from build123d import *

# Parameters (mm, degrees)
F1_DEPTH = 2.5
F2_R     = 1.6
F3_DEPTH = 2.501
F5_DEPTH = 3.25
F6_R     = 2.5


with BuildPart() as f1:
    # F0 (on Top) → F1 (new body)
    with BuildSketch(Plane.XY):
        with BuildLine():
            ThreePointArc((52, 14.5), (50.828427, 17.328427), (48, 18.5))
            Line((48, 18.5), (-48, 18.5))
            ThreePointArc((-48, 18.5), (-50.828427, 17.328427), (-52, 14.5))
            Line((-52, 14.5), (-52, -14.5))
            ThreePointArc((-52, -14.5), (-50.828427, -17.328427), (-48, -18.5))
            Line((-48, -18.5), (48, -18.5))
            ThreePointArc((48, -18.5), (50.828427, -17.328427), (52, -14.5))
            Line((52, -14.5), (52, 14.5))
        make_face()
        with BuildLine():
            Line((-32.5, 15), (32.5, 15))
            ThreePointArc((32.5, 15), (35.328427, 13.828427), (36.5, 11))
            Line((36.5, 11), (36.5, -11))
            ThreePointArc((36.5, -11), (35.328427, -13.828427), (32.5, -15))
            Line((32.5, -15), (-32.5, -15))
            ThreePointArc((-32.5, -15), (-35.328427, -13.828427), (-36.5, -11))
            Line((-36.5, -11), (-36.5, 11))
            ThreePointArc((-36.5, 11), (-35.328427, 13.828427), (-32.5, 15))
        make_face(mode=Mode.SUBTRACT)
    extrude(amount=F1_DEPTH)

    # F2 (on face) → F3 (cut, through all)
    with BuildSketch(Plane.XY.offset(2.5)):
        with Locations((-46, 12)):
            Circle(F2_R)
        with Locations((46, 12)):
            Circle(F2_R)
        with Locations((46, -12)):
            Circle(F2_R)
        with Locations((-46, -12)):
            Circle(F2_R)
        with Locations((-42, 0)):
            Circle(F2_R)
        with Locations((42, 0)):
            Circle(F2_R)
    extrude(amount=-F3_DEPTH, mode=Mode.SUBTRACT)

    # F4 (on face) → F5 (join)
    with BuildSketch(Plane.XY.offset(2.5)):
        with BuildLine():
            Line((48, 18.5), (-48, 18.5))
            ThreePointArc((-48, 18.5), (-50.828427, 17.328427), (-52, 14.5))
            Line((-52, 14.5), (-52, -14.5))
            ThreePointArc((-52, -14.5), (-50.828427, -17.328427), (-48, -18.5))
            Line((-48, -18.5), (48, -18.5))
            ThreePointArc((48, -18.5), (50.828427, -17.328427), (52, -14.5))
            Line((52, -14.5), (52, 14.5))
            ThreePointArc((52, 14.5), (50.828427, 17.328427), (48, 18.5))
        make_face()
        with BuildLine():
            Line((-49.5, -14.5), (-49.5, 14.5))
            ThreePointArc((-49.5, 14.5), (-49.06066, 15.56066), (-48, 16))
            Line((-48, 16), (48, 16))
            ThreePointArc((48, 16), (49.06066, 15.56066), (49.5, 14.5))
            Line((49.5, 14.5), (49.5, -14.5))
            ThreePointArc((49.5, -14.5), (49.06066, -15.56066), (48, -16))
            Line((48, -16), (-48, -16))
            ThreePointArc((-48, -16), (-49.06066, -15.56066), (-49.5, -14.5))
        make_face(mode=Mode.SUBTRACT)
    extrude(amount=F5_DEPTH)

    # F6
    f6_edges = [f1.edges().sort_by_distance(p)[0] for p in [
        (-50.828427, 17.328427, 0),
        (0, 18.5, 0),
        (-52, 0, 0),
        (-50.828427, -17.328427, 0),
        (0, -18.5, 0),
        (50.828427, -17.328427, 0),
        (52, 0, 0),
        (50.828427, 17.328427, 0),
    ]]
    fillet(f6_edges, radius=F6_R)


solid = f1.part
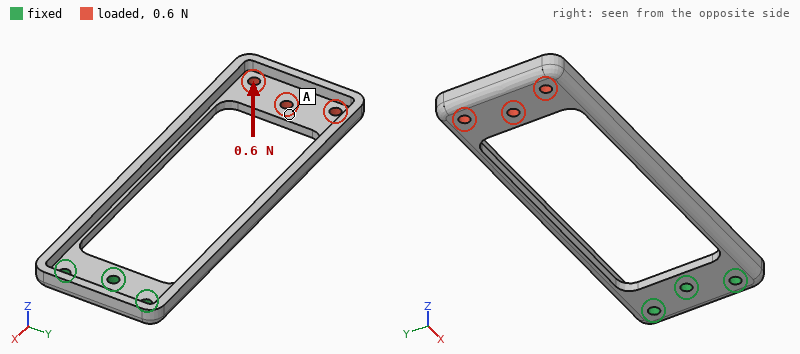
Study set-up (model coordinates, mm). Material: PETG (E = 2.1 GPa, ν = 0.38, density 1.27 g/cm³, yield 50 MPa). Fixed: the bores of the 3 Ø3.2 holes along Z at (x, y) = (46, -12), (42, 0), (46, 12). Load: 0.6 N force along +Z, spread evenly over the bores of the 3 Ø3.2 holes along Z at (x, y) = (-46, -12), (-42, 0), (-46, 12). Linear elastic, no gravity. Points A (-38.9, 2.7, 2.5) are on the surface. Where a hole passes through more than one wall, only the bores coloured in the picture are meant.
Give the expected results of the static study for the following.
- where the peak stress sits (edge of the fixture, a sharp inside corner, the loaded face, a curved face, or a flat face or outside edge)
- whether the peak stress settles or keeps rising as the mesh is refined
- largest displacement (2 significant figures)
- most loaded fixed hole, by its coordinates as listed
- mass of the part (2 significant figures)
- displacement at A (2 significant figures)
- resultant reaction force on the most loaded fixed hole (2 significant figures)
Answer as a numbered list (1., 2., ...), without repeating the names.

1. edge of the fixture
2. keeps rising
3. 1.0 mm
4. (42, 0)
5. 7.4 g
6. 0.82 mm
7. 0.58 N
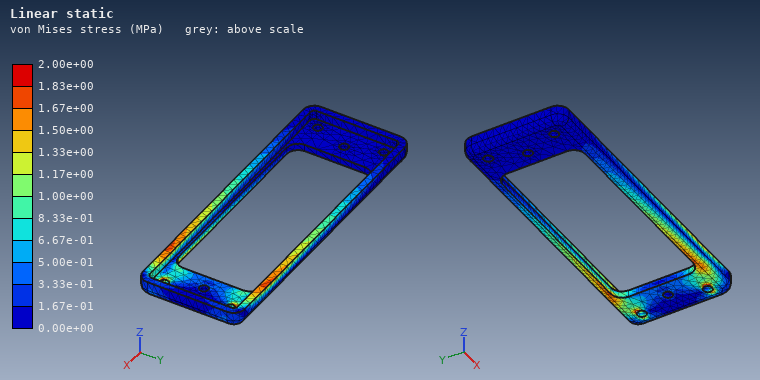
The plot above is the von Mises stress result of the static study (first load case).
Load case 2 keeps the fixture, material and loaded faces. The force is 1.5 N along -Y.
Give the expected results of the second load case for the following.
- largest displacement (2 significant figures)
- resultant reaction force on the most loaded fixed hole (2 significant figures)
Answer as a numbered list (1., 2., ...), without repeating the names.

1. 1.1 mm
2. 4.4 N
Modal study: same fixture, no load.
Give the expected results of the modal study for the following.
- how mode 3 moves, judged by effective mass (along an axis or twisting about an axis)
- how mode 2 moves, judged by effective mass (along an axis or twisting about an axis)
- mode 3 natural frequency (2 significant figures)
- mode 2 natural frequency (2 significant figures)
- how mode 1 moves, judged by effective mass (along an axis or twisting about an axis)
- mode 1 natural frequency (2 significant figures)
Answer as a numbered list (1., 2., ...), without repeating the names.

1. twisting about X
2. along Y
3. 210 Hz
4. 100 Hz
5. along Z
6. 76 Hz
